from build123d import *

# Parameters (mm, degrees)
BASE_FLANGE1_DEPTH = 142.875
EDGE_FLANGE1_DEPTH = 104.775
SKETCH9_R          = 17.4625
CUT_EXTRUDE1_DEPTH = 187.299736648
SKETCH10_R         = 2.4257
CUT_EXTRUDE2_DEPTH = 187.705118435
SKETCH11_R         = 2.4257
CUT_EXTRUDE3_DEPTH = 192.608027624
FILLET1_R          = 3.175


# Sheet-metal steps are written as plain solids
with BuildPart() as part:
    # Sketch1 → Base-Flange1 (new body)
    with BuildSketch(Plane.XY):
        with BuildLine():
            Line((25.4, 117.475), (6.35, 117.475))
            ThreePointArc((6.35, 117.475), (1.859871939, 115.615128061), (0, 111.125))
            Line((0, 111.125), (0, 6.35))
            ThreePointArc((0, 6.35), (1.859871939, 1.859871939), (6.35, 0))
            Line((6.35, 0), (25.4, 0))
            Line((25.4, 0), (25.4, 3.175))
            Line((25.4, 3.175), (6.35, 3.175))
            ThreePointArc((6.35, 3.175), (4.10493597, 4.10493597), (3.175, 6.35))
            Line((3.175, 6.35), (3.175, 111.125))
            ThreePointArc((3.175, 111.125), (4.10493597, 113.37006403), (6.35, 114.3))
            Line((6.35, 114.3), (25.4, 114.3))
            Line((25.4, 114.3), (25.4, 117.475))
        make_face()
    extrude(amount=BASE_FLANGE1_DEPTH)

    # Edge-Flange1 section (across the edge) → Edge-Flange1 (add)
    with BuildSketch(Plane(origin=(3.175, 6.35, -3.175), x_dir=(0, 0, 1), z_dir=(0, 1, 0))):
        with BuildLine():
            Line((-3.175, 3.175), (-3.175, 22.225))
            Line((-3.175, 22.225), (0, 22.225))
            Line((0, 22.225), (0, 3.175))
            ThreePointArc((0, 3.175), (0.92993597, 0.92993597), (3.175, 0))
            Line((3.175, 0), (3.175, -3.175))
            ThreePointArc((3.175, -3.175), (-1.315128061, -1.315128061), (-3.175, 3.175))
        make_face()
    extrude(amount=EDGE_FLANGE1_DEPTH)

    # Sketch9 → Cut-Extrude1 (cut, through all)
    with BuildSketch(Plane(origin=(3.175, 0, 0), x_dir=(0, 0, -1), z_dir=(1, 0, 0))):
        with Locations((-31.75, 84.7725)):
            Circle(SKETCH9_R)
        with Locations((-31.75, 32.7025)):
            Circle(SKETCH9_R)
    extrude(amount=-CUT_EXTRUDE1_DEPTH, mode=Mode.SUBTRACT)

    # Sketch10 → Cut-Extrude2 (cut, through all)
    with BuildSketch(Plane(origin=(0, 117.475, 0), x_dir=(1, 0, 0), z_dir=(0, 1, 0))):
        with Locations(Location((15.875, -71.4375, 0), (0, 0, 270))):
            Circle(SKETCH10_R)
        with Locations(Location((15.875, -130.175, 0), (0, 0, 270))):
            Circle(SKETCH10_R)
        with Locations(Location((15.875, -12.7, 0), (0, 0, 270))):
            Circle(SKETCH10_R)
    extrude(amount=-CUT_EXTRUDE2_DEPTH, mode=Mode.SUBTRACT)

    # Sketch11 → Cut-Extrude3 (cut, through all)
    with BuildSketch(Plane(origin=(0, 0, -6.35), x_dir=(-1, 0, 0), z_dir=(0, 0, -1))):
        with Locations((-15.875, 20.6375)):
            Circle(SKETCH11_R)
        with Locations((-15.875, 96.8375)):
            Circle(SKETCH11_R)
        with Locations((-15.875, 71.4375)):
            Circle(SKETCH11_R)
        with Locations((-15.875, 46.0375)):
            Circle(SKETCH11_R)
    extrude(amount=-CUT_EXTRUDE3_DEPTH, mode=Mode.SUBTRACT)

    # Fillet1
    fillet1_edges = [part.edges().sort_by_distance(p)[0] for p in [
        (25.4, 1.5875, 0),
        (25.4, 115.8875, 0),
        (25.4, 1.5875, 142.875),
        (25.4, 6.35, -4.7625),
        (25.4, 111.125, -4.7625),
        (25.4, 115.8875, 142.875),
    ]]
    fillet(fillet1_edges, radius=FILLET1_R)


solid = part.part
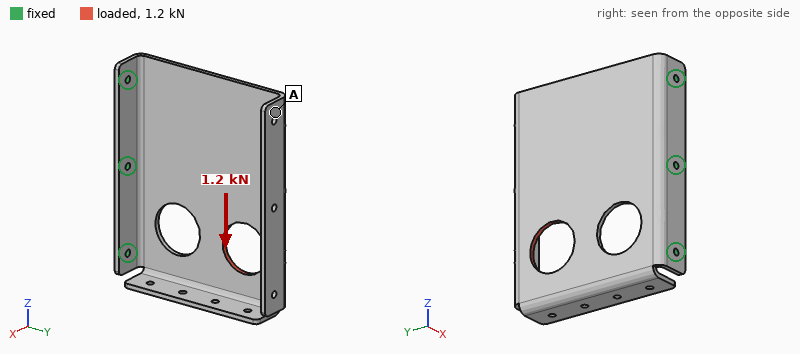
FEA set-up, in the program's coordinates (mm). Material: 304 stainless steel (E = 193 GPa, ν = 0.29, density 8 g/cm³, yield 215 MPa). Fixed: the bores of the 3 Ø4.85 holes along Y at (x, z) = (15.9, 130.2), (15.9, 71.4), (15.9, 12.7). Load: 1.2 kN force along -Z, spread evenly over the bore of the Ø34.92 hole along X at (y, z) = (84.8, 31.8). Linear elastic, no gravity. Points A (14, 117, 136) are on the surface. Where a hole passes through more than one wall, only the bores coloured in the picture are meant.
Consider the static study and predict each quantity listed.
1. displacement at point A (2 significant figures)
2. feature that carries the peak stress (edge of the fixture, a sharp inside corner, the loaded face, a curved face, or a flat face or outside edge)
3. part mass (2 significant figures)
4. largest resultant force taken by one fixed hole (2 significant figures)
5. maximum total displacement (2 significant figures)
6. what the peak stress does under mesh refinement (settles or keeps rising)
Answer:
0.16 mm
edge of the fixture
590 g
920 N
0.27 mm
keeps rising
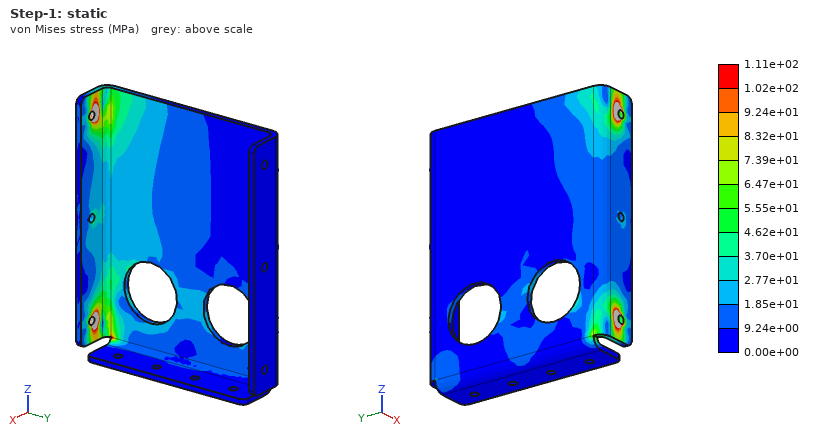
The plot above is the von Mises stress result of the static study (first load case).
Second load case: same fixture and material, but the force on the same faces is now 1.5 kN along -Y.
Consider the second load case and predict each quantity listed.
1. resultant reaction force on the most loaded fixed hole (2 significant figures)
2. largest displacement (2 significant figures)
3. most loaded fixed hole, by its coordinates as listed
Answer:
1000 N
0.49 mm
(15.9, 12.7)
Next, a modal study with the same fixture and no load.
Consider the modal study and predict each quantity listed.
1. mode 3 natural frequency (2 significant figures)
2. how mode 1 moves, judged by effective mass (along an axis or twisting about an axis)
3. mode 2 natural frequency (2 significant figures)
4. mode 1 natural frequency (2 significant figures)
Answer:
830 Hz
along X
270 Hz
120 Hz
